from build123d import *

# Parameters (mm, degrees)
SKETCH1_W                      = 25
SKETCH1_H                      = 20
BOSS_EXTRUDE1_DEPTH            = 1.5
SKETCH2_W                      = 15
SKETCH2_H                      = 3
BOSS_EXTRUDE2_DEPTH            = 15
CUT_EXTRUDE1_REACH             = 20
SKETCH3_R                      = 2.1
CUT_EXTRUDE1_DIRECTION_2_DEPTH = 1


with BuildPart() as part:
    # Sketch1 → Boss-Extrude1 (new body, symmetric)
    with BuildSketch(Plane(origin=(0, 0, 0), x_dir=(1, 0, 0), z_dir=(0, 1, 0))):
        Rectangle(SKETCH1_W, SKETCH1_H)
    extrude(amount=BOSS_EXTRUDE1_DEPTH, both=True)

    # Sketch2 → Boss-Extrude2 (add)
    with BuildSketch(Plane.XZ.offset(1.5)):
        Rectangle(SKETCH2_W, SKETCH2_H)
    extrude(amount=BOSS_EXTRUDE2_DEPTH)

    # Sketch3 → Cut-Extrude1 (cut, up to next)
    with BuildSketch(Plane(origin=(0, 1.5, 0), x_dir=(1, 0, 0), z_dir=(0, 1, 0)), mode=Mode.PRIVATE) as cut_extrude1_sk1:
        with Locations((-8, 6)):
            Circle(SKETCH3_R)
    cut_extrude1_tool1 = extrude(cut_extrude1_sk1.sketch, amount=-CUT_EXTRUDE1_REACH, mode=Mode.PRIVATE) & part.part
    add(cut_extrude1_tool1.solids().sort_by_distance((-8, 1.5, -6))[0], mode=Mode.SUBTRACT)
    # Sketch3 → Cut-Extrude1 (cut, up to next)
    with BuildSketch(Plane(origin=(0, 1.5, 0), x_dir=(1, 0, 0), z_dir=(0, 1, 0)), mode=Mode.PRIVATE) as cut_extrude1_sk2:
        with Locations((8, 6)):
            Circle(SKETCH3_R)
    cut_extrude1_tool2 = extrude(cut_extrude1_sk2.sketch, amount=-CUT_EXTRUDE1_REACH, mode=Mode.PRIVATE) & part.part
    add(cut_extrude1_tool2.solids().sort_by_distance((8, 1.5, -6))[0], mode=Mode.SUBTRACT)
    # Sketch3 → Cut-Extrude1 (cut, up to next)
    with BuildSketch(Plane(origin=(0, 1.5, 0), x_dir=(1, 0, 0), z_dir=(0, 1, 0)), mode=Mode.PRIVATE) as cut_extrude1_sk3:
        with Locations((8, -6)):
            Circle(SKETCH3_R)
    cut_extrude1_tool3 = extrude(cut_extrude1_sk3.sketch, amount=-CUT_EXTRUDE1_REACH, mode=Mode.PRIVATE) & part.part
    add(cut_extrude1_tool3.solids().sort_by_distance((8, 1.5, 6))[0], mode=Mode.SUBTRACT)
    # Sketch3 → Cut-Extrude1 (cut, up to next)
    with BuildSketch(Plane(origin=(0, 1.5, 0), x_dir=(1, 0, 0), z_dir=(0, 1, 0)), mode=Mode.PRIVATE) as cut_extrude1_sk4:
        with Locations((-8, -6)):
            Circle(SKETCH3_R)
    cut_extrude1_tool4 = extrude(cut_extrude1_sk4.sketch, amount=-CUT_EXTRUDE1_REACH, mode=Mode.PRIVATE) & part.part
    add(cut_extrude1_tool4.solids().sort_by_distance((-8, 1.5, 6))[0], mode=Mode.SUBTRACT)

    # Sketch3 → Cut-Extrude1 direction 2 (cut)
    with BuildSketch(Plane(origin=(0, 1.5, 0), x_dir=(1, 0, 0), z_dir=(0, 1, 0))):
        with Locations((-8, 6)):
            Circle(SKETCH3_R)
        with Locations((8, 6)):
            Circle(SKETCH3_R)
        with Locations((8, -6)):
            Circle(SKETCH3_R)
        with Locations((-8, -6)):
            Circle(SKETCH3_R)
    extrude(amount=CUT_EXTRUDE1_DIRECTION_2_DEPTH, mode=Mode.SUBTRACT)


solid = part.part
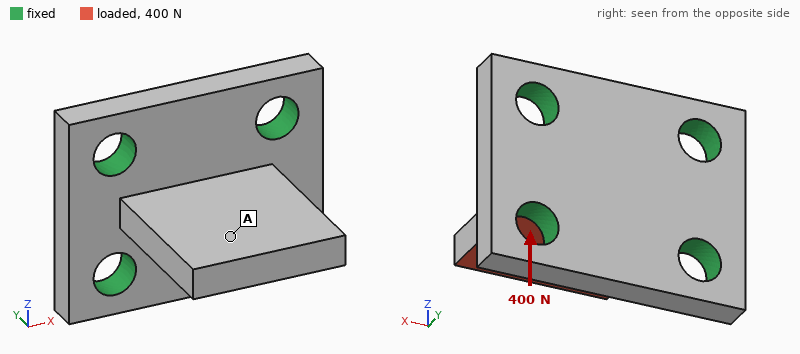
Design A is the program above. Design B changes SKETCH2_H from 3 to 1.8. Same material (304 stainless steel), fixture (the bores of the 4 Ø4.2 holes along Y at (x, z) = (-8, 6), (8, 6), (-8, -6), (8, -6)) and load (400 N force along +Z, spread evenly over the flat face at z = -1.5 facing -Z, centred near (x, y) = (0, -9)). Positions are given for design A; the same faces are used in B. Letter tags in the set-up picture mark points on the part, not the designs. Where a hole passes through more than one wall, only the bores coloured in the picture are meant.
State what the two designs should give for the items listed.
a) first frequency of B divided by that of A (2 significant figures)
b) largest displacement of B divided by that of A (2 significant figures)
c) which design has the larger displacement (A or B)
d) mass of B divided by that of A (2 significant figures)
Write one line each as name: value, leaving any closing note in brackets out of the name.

first frequency of B divided by that of A: 0.66
largest displacement of B divided by that of A: 3.9
which design has the larger displacement: B
mass of B divided by that of A: 0.87
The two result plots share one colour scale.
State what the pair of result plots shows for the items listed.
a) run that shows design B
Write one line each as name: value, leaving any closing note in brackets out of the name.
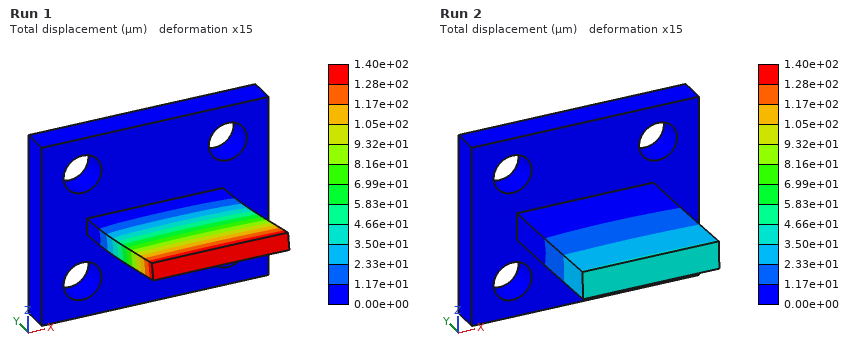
run that shows design B: Run 1
